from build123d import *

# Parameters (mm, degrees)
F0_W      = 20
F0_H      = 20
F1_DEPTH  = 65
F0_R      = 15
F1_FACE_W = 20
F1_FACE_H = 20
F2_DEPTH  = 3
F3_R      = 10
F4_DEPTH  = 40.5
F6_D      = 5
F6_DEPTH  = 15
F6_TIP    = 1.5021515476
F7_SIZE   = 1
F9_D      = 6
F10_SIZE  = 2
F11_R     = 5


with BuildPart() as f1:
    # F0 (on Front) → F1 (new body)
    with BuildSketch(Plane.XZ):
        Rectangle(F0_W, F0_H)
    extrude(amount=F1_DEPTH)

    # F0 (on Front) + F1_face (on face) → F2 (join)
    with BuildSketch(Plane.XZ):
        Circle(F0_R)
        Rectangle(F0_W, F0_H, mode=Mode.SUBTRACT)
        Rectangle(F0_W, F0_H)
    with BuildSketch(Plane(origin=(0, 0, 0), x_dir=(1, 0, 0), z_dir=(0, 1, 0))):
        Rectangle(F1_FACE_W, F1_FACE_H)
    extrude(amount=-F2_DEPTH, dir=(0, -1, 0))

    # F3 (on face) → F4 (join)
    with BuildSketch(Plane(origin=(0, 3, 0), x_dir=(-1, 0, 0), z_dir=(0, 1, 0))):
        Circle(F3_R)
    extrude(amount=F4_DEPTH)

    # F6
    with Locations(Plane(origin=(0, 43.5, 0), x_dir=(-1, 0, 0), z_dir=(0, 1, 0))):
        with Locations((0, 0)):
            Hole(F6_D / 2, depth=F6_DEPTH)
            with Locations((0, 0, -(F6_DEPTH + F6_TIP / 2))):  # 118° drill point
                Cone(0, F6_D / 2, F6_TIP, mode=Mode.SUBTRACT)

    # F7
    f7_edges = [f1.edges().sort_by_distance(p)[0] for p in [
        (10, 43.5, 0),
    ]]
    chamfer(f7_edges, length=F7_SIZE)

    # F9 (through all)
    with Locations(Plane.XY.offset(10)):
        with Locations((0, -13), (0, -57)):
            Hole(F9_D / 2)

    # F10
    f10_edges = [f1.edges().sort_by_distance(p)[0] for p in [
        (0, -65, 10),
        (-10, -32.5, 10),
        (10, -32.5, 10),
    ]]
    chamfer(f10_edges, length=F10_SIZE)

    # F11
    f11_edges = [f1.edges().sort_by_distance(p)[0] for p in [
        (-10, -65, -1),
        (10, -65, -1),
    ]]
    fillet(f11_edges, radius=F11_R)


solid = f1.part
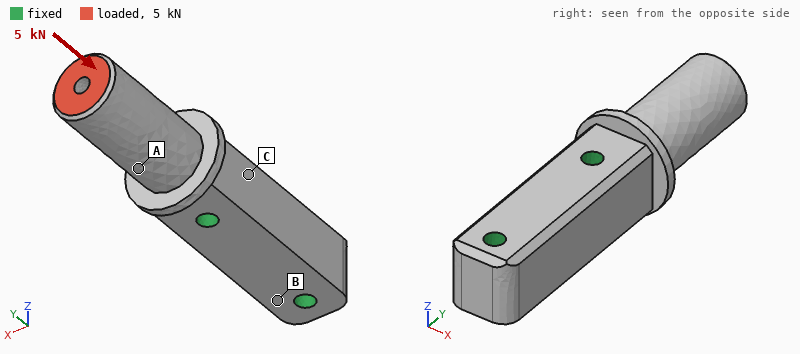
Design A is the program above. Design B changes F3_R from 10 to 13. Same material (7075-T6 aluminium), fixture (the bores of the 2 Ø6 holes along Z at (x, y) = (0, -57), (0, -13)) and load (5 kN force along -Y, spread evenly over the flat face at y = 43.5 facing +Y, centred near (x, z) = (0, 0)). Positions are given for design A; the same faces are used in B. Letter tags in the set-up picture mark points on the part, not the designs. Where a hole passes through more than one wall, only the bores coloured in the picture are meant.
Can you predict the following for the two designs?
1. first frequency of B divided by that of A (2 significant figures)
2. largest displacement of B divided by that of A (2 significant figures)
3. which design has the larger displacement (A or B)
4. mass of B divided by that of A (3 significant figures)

0.84
0.68
A
1.23
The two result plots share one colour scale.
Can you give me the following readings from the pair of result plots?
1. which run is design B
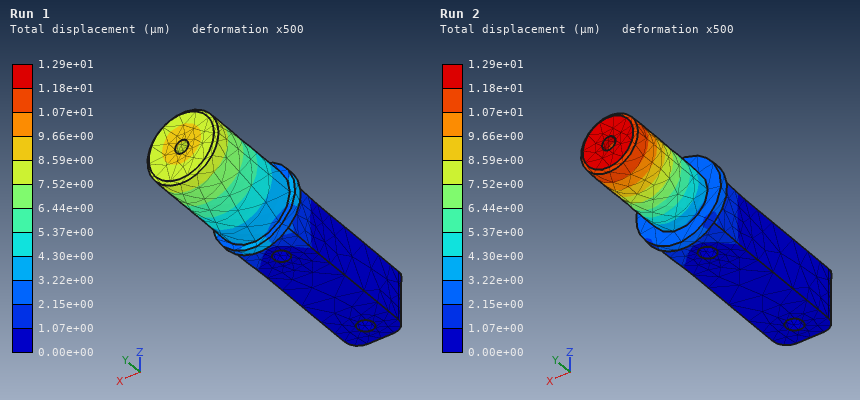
Run 1
